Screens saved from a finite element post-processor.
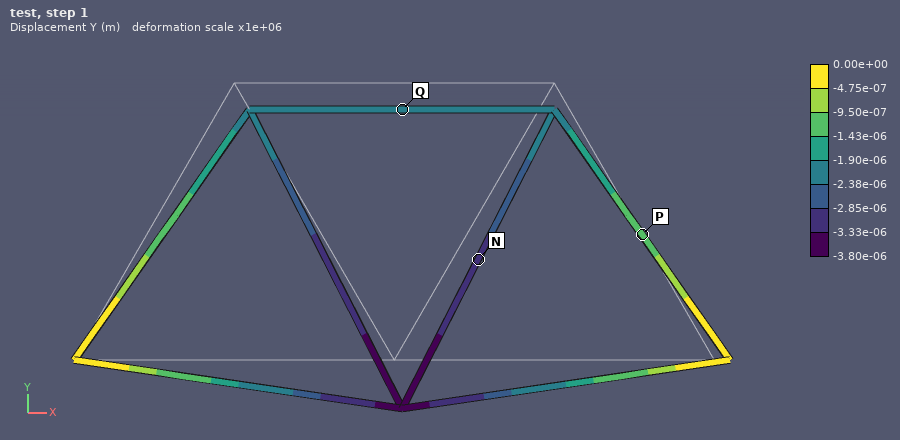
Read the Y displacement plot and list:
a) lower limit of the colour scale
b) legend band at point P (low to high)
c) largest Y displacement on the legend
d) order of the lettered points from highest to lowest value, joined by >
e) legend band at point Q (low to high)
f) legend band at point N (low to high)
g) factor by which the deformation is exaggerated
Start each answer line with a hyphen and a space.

- -3.80e-06 m
- -1.43e-06 to -9.50e-07 m
- 0.00e+00 m
- P > Q > N
- -2.38e-06 to -1.90e-06 m
- -3.33e-06 to -2.85e-06 m
- 1e+06
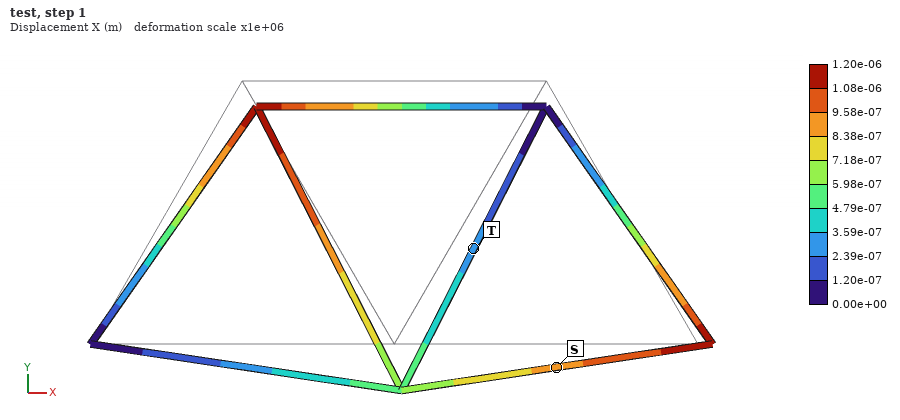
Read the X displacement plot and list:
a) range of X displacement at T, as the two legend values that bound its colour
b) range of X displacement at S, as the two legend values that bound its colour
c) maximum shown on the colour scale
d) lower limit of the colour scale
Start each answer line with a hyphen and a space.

- 2.39e-07 to 3.59e-07 m
- 8.38e-07 to 9.58e-07 m
- 1.20e-06 m
- 0.00e+00 m
